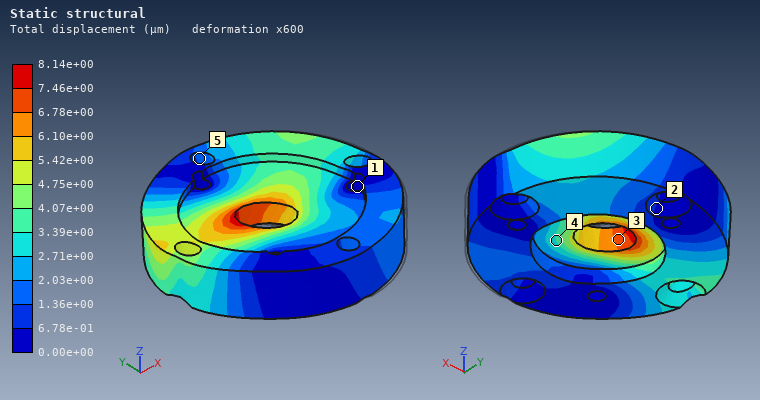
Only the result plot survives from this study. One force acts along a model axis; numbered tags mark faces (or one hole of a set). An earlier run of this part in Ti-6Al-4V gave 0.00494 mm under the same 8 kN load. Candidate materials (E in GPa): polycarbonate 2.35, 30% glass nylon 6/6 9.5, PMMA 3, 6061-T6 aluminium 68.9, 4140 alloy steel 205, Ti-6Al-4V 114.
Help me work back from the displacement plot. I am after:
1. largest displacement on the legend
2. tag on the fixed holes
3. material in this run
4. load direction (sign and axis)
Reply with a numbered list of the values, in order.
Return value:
1. 8.14e+00 µm
2. 1
3. 6061-T6 aluminium
4. -X
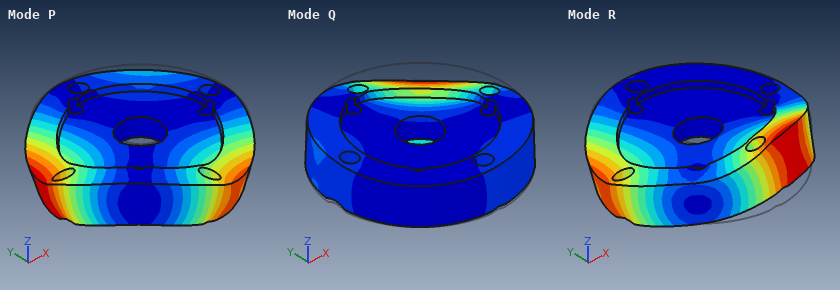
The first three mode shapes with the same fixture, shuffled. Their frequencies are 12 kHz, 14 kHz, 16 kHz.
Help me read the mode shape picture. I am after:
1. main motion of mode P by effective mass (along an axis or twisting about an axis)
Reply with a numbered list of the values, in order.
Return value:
1. along Z
